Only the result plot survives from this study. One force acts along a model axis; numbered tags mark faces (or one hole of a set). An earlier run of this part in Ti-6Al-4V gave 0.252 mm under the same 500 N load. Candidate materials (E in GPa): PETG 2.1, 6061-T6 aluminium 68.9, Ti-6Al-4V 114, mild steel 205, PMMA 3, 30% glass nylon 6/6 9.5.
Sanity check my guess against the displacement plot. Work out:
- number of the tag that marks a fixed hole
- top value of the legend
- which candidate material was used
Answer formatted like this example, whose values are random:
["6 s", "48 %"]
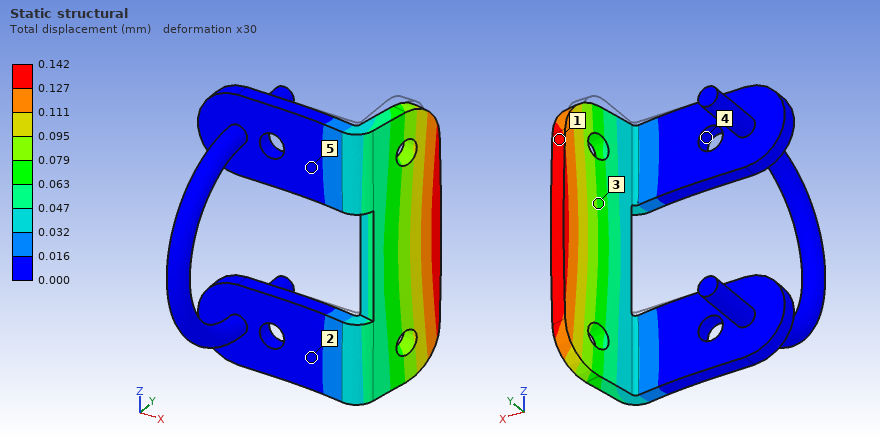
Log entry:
["4", "0.142 mm", "mild steel"]
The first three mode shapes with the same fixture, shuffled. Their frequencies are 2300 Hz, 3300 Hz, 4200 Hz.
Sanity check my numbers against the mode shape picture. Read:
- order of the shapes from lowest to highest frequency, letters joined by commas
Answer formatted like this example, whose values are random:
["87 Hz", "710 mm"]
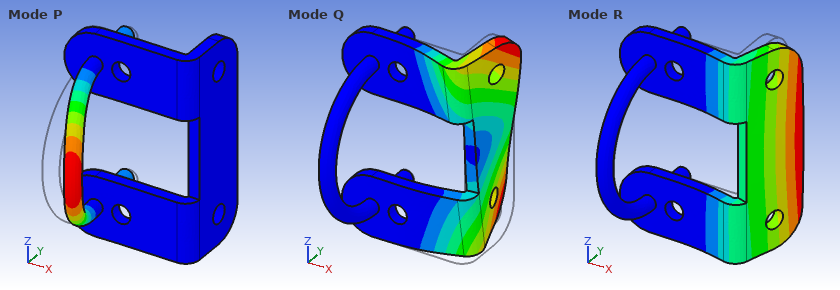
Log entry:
["R, P, Q"]
